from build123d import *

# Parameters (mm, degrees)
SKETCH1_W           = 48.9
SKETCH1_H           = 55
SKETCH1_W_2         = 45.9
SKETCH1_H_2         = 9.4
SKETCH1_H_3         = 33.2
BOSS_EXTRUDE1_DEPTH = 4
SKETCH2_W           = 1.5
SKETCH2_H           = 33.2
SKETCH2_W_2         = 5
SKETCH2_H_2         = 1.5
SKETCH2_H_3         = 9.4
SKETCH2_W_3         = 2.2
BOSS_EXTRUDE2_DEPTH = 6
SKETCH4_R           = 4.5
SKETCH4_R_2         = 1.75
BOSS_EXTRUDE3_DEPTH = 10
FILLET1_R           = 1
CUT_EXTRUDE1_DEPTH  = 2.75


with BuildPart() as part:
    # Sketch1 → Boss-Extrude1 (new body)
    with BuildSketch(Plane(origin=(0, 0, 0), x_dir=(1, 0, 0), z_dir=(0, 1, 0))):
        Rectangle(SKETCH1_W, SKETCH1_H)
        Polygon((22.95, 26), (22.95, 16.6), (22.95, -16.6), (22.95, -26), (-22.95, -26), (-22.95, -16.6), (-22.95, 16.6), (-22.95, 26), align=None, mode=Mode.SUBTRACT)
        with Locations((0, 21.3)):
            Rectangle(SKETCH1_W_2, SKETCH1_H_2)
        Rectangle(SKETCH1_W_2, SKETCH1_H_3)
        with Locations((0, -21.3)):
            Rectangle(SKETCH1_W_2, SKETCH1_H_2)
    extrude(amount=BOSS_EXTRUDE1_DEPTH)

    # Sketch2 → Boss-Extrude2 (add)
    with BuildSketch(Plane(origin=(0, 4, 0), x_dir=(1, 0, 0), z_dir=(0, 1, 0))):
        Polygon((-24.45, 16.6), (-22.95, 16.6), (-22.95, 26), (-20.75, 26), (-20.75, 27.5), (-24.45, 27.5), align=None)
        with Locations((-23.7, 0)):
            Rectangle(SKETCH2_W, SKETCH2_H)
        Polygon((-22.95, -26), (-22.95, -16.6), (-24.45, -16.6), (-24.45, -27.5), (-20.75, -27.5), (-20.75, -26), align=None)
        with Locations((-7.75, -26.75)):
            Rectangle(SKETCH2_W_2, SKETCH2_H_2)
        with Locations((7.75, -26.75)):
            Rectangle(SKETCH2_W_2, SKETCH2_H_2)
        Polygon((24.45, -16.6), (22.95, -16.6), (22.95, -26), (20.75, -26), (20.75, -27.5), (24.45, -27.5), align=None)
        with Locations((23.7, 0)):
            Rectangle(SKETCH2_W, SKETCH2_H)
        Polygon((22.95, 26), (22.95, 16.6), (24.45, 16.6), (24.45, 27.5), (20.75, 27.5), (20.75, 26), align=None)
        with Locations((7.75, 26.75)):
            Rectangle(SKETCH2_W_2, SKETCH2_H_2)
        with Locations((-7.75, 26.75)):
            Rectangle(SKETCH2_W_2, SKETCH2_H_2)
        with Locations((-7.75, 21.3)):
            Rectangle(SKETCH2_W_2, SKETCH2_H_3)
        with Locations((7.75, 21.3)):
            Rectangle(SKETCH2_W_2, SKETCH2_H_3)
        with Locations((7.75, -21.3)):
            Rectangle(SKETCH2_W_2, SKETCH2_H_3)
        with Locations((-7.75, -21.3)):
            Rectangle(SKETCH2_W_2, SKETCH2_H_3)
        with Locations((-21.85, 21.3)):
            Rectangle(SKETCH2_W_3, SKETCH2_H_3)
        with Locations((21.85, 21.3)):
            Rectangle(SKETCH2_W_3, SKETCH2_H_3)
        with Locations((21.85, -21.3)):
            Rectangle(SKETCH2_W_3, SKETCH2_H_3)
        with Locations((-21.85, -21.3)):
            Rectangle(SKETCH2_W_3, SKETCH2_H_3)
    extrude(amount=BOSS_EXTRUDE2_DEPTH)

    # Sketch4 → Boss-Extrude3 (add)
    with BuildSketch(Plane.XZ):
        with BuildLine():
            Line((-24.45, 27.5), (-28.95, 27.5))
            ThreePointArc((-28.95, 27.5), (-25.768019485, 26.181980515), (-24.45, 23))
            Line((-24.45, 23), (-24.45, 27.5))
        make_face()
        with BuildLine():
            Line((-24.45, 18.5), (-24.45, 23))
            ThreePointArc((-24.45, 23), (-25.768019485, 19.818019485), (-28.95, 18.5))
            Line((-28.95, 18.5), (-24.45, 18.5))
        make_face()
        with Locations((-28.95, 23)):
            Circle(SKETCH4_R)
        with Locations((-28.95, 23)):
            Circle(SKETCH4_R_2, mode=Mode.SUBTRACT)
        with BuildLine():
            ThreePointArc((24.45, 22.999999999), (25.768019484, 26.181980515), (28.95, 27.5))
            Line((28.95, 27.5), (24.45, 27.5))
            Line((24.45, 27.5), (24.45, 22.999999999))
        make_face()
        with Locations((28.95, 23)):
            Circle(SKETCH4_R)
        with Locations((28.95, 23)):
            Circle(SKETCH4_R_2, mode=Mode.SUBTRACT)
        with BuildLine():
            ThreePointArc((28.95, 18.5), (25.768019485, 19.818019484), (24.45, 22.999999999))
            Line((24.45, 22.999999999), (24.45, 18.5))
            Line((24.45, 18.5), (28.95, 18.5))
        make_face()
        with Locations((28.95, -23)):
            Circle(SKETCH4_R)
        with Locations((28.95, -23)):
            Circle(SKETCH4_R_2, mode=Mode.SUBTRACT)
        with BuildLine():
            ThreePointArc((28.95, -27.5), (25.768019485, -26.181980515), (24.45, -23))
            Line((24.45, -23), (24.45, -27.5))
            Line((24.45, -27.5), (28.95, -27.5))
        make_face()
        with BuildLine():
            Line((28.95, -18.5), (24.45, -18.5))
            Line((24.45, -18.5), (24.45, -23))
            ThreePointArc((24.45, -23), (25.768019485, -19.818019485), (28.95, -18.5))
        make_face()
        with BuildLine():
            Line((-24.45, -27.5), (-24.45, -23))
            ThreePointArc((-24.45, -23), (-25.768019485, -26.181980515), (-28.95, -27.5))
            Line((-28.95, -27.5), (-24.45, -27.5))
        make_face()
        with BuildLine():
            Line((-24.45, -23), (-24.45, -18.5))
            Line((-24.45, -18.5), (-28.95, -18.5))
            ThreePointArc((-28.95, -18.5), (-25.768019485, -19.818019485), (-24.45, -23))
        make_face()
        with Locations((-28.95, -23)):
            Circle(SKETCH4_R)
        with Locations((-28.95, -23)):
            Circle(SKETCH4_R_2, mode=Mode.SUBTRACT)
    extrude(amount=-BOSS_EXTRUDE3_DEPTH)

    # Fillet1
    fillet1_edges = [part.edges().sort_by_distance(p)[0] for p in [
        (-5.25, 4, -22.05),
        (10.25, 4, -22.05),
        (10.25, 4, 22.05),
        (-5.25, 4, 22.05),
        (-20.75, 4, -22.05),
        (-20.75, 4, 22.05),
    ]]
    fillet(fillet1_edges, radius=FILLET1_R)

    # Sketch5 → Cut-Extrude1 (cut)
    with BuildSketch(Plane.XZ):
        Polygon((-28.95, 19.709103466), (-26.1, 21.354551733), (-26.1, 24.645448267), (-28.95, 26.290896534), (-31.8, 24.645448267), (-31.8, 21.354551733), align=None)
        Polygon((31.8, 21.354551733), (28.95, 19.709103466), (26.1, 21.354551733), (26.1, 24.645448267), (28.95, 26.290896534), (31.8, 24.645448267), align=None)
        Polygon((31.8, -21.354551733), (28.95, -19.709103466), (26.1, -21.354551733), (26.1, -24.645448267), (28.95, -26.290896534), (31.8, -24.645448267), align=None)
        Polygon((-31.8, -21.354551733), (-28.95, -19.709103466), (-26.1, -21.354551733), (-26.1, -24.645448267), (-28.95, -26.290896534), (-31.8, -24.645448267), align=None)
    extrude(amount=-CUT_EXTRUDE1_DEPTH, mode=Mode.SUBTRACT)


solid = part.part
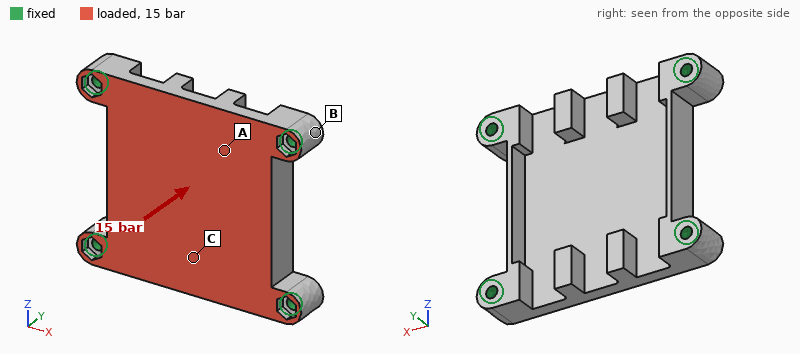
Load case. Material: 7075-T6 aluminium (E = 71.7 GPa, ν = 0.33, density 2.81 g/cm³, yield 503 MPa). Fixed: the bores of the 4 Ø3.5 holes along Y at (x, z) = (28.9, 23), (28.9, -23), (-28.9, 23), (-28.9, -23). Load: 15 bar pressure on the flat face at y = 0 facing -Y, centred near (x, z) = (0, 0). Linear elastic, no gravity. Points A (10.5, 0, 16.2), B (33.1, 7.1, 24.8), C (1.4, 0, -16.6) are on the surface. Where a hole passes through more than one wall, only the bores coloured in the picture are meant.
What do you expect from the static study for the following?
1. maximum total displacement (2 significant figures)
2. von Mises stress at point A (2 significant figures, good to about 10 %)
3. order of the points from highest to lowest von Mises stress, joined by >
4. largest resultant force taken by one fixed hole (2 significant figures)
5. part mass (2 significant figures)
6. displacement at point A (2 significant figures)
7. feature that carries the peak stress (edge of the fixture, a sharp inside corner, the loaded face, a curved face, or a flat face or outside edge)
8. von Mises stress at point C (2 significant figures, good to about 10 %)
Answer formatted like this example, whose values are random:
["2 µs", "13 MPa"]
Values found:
["0.11 mm", "42 MPa", "C > A > B", "1.5 kN", "45 g", "0.068 mm", "a curved face", "73 MPa"]
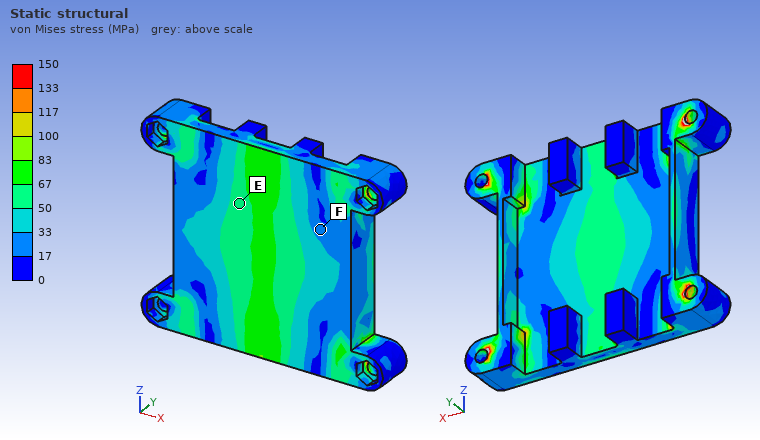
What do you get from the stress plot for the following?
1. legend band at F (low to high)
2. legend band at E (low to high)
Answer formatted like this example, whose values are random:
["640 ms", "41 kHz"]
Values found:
["17 to 33 MPa", "50 to 67 MPa"]
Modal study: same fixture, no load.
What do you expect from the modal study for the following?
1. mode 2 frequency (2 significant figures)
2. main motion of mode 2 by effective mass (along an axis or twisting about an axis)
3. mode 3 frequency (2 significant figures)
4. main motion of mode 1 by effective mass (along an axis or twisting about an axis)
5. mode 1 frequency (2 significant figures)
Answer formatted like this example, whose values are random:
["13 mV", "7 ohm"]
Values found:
["8300 Hz", "twisting about X", "11 kHz", "along Y", "6300 Hz"]
